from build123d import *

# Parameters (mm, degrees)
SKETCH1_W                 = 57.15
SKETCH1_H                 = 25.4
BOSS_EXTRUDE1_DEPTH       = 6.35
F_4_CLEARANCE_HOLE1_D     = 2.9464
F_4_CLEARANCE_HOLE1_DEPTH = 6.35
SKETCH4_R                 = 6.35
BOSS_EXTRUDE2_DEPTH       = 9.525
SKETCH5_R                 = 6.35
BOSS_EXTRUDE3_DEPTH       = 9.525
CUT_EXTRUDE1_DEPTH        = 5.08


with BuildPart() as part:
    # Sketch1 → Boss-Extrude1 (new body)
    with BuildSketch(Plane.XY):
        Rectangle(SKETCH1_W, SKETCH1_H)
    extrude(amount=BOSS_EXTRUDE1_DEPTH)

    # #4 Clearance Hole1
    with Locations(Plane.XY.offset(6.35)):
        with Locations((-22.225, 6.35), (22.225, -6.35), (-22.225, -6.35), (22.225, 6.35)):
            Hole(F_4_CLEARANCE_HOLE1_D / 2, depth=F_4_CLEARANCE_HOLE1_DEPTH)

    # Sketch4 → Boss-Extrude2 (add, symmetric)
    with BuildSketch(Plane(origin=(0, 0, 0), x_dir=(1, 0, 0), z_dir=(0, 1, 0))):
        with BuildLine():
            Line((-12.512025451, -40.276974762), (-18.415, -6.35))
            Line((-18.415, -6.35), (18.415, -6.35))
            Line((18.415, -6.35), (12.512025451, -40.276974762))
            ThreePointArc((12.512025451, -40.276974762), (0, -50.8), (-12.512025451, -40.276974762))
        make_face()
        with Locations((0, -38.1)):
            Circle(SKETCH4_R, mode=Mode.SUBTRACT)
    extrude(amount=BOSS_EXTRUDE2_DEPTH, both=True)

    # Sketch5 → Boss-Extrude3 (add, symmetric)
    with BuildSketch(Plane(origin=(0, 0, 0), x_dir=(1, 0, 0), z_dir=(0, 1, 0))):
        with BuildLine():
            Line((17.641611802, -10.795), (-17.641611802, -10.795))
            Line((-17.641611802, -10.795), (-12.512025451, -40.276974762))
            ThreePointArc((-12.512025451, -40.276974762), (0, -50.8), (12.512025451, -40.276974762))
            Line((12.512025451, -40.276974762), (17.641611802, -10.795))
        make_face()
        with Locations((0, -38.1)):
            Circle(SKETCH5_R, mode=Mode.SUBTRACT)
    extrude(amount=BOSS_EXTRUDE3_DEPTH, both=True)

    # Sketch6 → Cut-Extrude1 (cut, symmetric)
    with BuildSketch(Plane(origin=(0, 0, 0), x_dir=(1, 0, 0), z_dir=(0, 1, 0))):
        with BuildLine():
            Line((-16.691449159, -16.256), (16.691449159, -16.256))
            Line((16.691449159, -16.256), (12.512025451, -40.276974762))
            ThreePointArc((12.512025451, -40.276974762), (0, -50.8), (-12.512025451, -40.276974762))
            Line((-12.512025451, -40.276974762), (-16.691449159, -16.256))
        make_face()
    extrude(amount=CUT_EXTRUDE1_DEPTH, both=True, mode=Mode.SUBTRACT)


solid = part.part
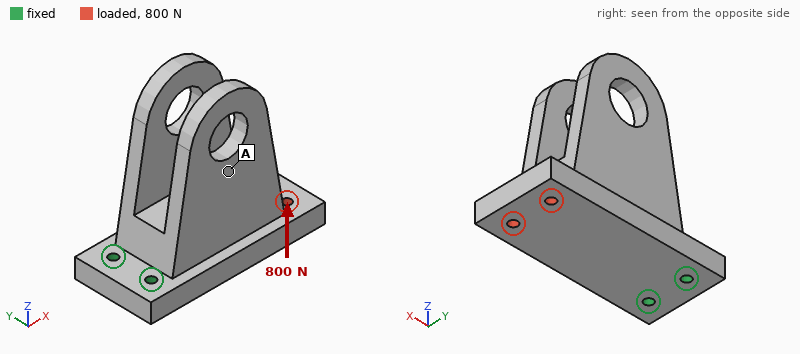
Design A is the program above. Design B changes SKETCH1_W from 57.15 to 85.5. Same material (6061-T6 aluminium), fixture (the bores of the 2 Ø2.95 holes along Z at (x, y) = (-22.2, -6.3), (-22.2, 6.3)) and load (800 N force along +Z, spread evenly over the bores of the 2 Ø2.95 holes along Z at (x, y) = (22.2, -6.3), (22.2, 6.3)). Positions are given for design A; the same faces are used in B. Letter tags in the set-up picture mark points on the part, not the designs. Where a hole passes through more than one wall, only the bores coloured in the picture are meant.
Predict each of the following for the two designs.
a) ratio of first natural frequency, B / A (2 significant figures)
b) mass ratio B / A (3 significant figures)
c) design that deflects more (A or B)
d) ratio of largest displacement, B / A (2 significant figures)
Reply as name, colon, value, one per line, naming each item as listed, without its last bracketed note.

ratio of first natural frequency, B / A: 0.84
mass ratio B / A: 1.20
design that deflects more: B
ratio of largest displacement, B / A: 1.2
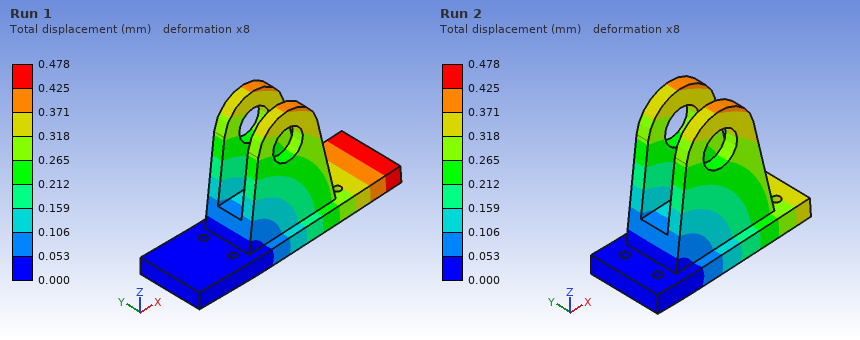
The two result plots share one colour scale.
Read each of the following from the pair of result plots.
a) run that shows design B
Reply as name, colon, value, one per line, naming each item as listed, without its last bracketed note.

run that shows design B: Run 1
